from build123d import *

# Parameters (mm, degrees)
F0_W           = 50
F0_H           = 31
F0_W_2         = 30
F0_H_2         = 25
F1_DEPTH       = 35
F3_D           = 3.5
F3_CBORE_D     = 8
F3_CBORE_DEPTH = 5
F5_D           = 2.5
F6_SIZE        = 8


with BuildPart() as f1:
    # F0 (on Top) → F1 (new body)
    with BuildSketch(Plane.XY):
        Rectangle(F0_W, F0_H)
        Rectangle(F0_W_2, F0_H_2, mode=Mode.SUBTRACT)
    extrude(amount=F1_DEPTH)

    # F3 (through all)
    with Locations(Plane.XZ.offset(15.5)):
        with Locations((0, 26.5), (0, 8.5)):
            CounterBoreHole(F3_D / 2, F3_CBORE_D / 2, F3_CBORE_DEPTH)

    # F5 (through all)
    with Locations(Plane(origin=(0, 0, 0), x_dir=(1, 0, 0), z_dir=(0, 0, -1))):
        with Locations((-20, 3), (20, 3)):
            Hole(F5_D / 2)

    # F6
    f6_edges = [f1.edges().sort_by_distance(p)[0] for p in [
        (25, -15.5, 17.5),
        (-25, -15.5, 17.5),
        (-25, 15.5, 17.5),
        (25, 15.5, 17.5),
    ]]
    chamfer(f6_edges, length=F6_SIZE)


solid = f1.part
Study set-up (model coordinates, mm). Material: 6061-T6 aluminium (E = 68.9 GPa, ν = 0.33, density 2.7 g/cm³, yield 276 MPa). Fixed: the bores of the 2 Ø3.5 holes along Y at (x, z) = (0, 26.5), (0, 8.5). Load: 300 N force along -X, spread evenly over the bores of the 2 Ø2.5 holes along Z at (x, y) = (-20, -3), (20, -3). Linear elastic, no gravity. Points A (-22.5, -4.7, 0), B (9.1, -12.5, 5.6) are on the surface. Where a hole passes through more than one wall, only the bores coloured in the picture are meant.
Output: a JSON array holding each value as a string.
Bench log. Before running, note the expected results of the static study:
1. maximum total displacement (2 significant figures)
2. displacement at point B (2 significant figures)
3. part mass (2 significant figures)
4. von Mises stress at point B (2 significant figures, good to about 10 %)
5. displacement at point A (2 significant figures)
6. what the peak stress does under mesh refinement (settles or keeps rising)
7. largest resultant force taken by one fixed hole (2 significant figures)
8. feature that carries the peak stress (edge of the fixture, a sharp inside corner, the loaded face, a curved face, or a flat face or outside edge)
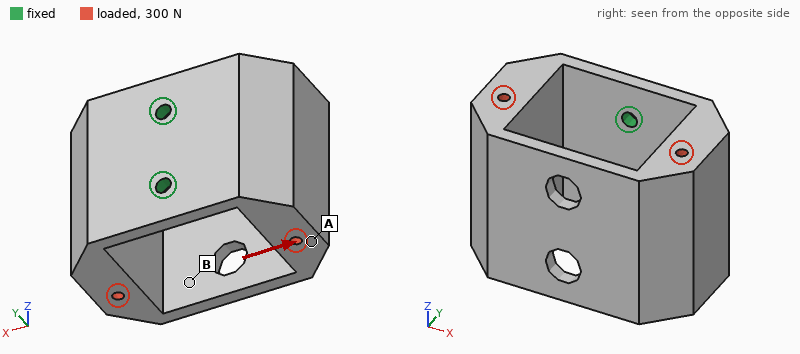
["0.16 mm", "0.14 mm", "62 g", "15 MPa", "0.13 mm", "keeps rising", "150 N", "edge of the fixture"]
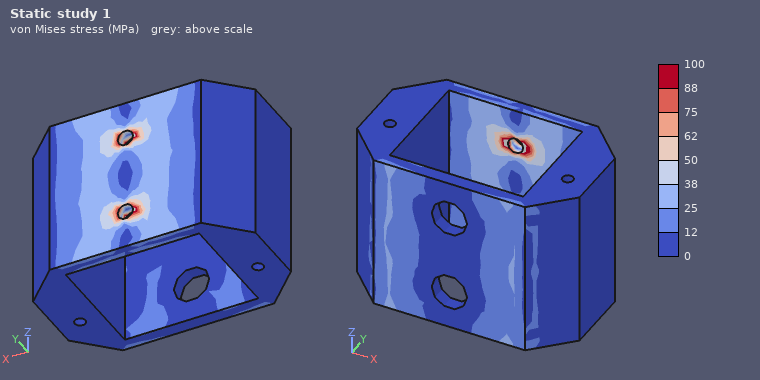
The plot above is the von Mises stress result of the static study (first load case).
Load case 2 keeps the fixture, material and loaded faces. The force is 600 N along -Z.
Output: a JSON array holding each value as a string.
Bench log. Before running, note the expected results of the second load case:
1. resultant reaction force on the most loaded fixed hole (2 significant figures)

["540 N"]
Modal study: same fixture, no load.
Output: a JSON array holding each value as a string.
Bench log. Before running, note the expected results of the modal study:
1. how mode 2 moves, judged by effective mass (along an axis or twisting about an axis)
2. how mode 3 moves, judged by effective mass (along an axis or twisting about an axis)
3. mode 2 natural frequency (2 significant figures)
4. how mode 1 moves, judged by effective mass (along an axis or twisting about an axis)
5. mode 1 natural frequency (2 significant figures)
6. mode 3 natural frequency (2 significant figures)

["along Z", "along Y", "1900 Hz", "along X", "980 Hz", "3500 Hz"]
